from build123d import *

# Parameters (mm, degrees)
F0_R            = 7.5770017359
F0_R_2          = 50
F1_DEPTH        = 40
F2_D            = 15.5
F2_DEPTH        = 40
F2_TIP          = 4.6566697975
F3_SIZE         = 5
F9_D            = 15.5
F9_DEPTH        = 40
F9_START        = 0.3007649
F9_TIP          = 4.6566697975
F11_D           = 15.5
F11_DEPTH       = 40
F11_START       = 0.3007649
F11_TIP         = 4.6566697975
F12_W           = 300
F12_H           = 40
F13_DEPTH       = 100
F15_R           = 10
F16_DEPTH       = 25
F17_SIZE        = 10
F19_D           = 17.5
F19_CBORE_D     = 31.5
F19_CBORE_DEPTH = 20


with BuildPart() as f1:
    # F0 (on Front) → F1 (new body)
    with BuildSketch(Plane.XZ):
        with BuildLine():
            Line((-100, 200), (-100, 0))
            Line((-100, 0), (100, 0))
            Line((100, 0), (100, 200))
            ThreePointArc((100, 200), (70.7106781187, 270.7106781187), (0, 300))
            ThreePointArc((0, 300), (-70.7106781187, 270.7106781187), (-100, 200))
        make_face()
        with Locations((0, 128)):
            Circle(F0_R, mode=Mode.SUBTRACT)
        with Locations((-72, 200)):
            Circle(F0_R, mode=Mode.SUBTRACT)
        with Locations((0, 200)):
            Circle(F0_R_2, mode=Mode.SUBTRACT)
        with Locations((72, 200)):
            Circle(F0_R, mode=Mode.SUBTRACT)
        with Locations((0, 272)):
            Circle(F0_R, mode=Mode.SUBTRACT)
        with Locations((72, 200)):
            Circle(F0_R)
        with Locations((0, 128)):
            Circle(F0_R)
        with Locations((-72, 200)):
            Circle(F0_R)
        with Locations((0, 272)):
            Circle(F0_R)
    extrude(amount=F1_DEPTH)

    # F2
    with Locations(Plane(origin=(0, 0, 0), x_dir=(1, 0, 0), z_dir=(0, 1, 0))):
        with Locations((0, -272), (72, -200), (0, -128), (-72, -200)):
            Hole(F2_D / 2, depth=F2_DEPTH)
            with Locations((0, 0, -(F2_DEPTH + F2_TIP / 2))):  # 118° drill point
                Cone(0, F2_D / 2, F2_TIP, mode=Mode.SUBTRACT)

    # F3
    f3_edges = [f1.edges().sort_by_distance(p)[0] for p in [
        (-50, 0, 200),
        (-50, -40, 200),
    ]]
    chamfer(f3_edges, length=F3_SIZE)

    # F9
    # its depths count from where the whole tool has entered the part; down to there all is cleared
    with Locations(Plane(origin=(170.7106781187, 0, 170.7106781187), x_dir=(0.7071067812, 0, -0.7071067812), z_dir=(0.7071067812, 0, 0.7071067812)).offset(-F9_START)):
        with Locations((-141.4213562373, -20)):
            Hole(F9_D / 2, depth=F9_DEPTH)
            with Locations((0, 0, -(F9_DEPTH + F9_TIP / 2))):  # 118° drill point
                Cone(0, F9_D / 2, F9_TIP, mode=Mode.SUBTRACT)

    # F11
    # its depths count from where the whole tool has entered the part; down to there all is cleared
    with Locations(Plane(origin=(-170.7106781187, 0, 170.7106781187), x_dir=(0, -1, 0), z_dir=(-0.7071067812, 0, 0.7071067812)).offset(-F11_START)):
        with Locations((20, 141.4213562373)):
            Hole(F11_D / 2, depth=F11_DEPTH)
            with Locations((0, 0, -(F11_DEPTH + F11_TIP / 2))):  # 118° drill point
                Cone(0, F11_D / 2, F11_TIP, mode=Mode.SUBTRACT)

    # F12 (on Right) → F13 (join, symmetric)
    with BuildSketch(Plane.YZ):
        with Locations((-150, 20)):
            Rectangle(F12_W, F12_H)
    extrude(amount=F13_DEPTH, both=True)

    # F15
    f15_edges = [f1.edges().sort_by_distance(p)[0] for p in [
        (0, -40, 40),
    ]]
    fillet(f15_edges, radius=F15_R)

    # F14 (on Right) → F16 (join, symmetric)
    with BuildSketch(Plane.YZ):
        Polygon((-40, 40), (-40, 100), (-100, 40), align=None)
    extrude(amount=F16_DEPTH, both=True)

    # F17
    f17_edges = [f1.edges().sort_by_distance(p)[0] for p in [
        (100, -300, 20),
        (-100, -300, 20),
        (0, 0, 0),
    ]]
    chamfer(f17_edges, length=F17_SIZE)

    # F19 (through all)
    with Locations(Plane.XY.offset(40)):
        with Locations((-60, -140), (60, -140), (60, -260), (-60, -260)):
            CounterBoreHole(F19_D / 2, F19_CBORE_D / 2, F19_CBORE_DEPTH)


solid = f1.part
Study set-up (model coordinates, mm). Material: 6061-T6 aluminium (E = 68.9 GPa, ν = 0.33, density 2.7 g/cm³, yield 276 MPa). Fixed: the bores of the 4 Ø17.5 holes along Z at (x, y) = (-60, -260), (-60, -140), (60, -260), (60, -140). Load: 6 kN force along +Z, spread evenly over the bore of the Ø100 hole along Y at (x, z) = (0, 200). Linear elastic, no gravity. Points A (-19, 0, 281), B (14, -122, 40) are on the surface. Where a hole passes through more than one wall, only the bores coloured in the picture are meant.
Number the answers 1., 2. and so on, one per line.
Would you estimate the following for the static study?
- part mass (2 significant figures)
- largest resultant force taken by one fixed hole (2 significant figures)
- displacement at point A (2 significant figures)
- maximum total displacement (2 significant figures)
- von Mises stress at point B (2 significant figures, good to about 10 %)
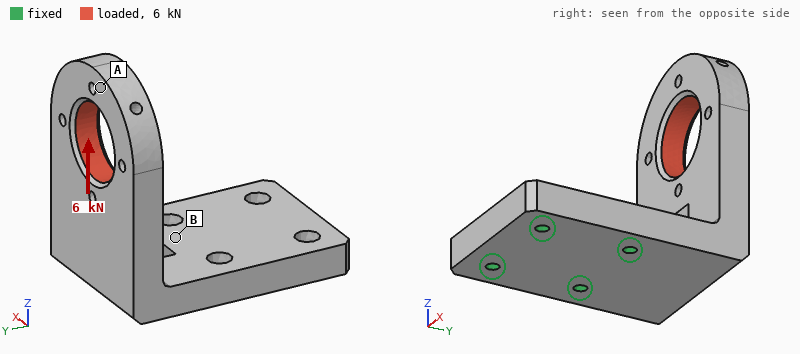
1. 11 kg
2. 6.2 kN
3. 0.22 mm
4. 0.24 mm
5. 12 MPa
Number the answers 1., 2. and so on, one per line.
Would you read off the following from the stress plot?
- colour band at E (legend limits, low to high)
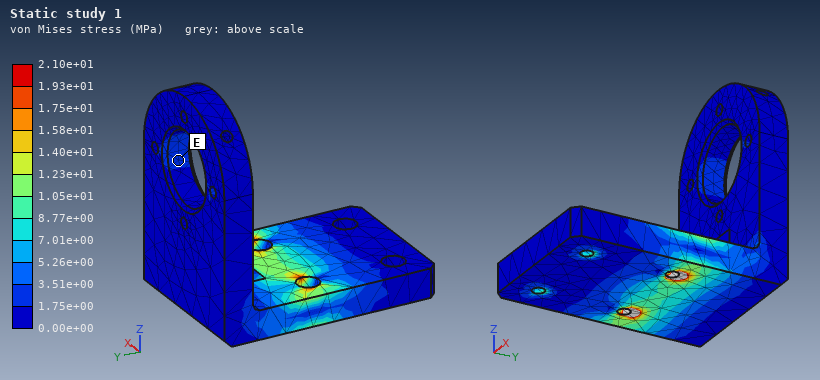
1. 1.75e+00 to 3.51e+00 MPa
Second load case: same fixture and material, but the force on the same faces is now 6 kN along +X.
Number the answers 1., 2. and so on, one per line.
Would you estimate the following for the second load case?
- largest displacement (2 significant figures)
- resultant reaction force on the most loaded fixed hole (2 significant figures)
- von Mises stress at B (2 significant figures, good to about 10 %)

1. 0.21 mm
2. 12 kN
3. 9.3 MPa
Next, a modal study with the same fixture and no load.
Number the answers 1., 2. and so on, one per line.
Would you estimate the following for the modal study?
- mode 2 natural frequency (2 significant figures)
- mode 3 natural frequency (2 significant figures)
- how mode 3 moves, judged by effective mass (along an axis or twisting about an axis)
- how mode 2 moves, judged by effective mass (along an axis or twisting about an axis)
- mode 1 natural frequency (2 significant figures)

1. 580 Hz
2. 980 Hz
3. along Z
4. along X
5. 330 Hz
